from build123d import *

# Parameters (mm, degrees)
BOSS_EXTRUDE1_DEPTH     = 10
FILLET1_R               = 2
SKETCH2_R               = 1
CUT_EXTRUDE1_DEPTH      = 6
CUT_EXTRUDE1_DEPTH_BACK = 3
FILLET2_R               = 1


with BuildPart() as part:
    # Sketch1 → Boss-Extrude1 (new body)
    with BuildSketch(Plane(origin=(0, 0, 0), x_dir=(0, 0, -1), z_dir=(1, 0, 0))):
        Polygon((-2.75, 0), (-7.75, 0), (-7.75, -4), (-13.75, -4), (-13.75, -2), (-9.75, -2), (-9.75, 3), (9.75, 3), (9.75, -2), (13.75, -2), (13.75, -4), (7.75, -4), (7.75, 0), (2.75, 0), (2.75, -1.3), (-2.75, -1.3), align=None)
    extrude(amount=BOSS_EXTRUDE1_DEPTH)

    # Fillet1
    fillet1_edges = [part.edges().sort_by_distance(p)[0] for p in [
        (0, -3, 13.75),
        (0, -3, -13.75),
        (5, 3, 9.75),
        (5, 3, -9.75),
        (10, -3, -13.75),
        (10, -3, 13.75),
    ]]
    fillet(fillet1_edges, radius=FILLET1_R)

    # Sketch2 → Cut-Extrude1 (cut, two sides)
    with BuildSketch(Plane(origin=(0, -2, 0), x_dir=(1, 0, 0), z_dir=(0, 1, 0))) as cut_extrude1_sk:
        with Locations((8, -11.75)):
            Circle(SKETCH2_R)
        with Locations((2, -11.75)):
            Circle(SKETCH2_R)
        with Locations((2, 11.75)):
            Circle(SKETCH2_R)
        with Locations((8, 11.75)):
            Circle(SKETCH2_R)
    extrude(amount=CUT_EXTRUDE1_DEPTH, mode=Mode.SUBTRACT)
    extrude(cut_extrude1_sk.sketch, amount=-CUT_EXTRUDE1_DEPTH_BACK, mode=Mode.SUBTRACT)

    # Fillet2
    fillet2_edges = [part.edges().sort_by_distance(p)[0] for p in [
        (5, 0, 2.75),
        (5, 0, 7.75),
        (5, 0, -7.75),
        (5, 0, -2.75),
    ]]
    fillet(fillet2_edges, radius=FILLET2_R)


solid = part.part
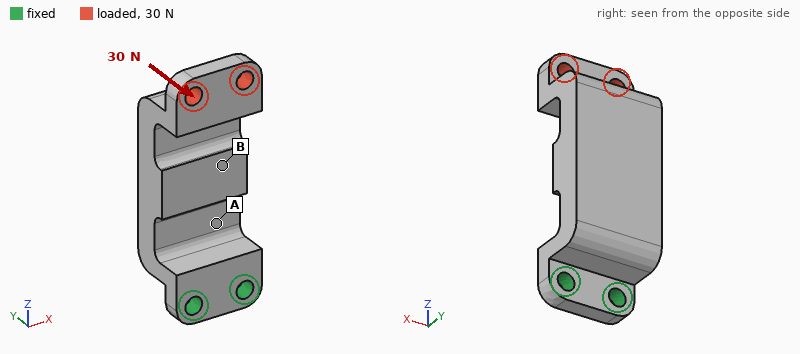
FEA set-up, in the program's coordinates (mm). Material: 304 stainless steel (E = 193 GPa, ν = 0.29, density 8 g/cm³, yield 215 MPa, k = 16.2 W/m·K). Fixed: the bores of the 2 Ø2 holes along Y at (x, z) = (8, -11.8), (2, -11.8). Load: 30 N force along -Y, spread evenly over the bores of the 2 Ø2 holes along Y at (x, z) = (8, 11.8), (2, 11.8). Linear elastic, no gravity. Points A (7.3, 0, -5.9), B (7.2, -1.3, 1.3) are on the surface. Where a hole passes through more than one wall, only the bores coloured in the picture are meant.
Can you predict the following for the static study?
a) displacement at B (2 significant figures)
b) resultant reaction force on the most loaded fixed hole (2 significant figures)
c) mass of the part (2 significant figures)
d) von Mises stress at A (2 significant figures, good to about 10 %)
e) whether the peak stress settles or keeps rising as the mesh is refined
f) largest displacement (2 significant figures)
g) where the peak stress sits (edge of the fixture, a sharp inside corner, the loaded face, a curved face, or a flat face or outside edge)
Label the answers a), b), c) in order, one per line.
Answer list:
a) 32 µm
b) 16 N
c) 7.5 g
d) 34 MPa
e) keeps rising
f) 78 µm
g) edge of the fixture
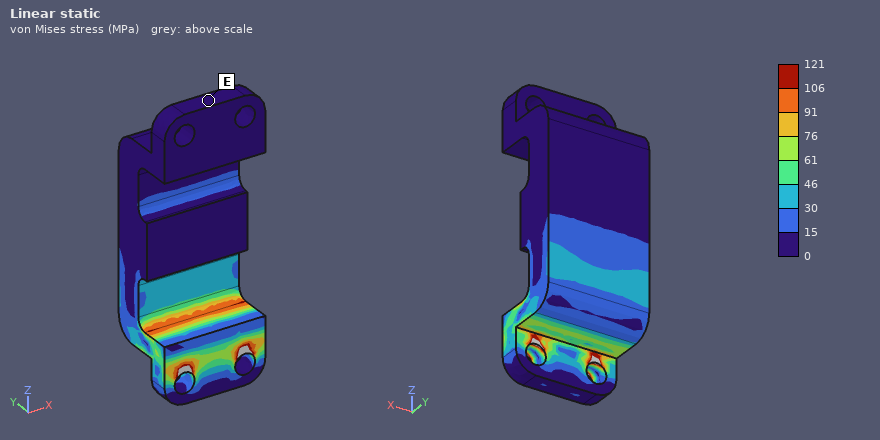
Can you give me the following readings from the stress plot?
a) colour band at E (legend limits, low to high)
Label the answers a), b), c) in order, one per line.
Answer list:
a) 0 to 15 MPa
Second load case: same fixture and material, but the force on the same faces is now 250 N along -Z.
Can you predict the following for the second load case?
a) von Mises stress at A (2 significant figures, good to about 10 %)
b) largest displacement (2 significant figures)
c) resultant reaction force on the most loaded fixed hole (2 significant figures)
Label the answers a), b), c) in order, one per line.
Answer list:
a) 80 MPa
b) 81 µm
c) 130 N
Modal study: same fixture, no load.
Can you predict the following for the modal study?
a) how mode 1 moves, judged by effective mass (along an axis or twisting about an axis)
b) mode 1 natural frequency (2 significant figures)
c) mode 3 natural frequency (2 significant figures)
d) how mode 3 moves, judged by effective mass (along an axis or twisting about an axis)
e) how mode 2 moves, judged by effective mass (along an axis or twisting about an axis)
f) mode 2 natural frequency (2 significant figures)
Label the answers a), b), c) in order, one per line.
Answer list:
a) along Y
b) 2200 Hz
c) 13 kHz
d) along Z
e) along X
f) 5100 Hz
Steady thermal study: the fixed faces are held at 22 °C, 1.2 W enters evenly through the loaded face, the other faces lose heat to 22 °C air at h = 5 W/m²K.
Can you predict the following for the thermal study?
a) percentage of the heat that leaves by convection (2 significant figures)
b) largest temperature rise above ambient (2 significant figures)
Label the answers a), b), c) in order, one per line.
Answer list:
a) 13 %
b) 76 K
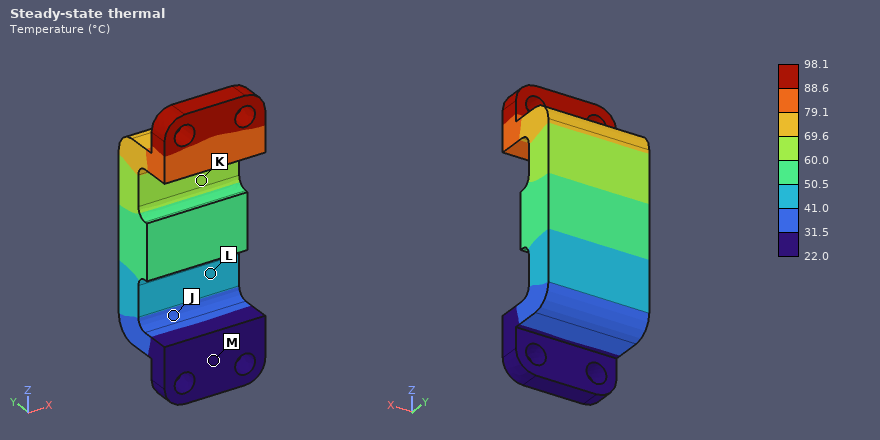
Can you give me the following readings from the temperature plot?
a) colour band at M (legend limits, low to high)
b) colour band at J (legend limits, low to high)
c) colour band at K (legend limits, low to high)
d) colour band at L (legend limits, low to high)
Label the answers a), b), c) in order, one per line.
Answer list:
a) 22.0 to 31.5 °C
b) 31.5 to 41.0 °C
c) 60.0 to 69.6 °C
d) 41.0 to 50.5 °C
